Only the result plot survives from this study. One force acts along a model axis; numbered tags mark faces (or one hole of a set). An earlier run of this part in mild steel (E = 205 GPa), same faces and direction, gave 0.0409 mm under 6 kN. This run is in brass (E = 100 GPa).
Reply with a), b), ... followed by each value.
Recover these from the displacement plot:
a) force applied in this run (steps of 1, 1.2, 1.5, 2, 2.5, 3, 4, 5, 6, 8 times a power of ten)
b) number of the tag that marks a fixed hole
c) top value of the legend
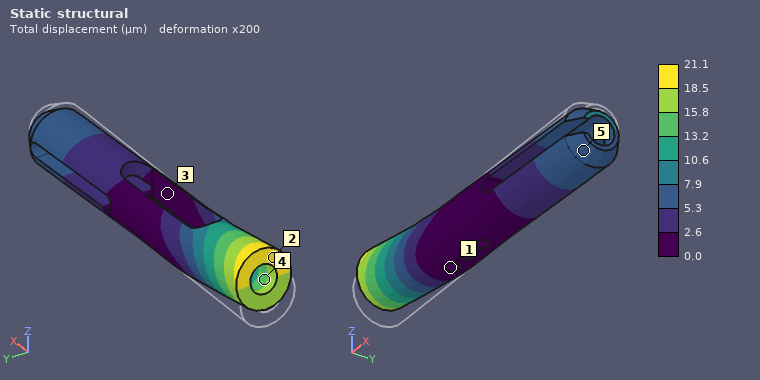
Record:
a) 1.5 kN
b) 1
c) 21.1 µm
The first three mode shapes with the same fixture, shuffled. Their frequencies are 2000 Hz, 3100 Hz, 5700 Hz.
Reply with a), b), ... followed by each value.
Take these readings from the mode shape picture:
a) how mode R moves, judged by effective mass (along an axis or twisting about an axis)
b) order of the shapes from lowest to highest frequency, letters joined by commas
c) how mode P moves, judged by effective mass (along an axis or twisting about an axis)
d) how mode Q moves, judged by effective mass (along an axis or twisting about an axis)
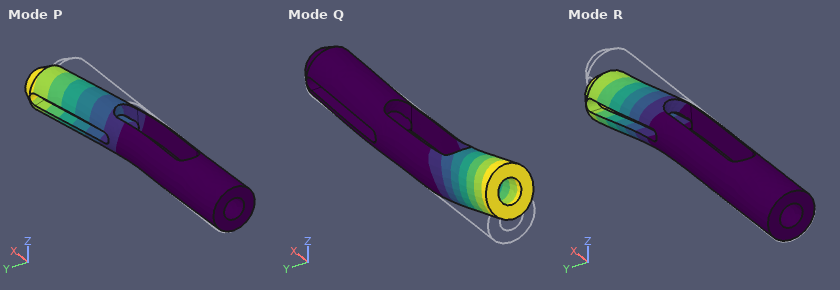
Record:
a) along Z
b) R, P, Q
c) along Y
d) along Z
